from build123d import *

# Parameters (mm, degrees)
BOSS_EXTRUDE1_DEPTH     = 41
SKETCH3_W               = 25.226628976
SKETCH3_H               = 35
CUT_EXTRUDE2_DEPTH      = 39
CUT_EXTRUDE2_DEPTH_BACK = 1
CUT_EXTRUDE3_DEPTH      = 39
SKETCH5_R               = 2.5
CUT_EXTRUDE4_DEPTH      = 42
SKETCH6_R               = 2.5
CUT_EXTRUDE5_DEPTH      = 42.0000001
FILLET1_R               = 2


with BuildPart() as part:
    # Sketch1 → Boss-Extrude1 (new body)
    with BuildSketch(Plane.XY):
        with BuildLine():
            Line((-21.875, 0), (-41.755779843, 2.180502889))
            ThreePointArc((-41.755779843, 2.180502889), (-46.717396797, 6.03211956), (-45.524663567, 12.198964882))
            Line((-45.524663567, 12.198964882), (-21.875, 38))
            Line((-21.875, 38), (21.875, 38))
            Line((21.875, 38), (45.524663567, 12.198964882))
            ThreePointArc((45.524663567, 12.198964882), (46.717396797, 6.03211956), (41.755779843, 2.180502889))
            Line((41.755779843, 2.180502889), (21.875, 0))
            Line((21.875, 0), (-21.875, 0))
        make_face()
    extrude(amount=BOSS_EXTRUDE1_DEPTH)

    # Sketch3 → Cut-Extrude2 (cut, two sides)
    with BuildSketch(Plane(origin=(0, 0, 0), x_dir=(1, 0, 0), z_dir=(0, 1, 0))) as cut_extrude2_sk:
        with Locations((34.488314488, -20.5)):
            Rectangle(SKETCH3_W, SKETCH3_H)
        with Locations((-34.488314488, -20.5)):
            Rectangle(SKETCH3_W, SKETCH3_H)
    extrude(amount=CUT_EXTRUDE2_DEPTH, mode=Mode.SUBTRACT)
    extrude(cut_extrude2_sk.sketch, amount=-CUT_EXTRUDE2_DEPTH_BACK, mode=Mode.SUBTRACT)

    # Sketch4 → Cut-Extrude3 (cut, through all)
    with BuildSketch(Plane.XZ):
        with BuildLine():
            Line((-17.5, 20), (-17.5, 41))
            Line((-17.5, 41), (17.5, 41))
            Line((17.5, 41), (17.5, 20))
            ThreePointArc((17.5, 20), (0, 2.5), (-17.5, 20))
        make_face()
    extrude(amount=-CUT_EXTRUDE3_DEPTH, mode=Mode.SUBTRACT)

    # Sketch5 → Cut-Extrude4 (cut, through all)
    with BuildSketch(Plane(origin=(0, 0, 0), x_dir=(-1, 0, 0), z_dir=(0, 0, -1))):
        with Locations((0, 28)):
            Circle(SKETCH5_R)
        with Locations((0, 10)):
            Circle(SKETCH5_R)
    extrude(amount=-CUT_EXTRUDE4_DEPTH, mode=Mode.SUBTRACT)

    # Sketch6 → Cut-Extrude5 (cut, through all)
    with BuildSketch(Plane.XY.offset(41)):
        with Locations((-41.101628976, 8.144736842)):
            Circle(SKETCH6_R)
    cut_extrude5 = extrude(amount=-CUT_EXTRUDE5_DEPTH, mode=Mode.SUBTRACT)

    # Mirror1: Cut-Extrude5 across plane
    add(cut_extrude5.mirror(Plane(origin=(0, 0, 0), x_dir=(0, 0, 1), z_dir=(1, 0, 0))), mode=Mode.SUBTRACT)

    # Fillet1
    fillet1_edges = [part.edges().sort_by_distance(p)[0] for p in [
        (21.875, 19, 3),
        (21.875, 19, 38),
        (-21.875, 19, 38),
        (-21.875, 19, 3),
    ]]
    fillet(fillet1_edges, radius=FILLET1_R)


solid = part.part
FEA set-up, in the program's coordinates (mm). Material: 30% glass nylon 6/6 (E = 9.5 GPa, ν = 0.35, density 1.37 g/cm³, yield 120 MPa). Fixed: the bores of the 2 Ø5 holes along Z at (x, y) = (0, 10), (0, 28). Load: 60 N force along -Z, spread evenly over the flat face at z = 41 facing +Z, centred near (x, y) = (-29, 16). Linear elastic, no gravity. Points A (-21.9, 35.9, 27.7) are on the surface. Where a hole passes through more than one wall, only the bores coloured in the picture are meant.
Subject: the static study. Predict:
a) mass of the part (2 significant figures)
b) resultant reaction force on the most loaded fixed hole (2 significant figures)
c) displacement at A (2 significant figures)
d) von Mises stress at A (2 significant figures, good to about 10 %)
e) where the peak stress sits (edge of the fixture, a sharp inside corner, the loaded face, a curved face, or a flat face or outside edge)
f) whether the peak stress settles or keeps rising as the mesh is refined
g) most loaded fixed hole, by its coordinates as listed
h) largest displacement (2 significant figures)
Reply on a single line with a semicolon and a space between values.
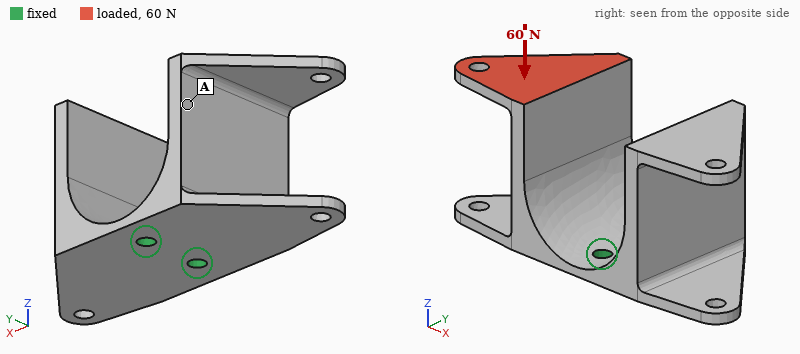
39 g; 39 N; 0.42 mm; 3.9 MPa; edge of the fixture; keeps rising; (0, 10); 1.0 mm
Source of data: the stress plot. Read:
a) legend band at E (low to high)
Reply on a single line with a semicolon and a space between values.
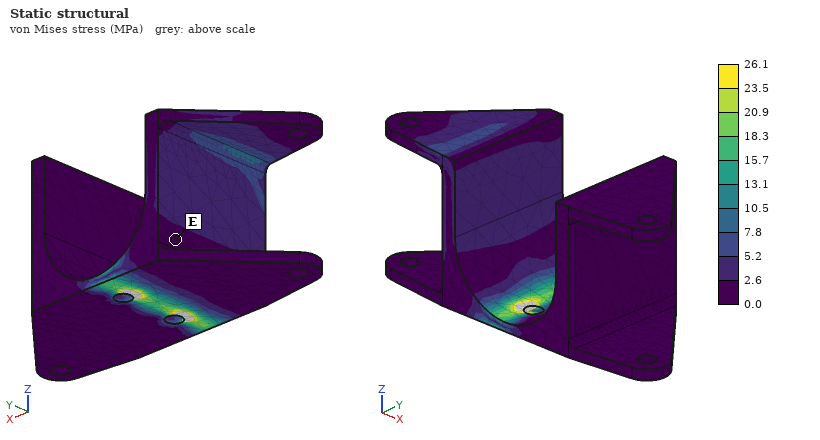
0.0 to 2.6 MPa
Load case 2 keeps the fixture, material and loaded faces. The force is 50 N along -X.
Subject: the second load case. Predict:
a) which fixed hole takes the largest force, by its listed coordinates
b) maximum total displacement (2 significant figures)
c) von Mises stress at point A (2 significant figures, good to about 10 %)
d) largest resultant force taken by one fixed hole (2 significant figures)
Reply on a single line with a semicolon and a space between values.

(0, 10); 1.3 mm; 5.4 MPa; 34 N
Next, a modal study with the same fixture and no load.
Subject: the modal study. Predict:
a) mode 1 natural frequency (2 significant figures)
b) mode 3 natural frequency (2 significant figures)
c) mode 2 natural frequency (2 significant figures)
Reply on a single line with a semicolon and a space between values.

430 Hz; 1300 Hz; 440 Hz
